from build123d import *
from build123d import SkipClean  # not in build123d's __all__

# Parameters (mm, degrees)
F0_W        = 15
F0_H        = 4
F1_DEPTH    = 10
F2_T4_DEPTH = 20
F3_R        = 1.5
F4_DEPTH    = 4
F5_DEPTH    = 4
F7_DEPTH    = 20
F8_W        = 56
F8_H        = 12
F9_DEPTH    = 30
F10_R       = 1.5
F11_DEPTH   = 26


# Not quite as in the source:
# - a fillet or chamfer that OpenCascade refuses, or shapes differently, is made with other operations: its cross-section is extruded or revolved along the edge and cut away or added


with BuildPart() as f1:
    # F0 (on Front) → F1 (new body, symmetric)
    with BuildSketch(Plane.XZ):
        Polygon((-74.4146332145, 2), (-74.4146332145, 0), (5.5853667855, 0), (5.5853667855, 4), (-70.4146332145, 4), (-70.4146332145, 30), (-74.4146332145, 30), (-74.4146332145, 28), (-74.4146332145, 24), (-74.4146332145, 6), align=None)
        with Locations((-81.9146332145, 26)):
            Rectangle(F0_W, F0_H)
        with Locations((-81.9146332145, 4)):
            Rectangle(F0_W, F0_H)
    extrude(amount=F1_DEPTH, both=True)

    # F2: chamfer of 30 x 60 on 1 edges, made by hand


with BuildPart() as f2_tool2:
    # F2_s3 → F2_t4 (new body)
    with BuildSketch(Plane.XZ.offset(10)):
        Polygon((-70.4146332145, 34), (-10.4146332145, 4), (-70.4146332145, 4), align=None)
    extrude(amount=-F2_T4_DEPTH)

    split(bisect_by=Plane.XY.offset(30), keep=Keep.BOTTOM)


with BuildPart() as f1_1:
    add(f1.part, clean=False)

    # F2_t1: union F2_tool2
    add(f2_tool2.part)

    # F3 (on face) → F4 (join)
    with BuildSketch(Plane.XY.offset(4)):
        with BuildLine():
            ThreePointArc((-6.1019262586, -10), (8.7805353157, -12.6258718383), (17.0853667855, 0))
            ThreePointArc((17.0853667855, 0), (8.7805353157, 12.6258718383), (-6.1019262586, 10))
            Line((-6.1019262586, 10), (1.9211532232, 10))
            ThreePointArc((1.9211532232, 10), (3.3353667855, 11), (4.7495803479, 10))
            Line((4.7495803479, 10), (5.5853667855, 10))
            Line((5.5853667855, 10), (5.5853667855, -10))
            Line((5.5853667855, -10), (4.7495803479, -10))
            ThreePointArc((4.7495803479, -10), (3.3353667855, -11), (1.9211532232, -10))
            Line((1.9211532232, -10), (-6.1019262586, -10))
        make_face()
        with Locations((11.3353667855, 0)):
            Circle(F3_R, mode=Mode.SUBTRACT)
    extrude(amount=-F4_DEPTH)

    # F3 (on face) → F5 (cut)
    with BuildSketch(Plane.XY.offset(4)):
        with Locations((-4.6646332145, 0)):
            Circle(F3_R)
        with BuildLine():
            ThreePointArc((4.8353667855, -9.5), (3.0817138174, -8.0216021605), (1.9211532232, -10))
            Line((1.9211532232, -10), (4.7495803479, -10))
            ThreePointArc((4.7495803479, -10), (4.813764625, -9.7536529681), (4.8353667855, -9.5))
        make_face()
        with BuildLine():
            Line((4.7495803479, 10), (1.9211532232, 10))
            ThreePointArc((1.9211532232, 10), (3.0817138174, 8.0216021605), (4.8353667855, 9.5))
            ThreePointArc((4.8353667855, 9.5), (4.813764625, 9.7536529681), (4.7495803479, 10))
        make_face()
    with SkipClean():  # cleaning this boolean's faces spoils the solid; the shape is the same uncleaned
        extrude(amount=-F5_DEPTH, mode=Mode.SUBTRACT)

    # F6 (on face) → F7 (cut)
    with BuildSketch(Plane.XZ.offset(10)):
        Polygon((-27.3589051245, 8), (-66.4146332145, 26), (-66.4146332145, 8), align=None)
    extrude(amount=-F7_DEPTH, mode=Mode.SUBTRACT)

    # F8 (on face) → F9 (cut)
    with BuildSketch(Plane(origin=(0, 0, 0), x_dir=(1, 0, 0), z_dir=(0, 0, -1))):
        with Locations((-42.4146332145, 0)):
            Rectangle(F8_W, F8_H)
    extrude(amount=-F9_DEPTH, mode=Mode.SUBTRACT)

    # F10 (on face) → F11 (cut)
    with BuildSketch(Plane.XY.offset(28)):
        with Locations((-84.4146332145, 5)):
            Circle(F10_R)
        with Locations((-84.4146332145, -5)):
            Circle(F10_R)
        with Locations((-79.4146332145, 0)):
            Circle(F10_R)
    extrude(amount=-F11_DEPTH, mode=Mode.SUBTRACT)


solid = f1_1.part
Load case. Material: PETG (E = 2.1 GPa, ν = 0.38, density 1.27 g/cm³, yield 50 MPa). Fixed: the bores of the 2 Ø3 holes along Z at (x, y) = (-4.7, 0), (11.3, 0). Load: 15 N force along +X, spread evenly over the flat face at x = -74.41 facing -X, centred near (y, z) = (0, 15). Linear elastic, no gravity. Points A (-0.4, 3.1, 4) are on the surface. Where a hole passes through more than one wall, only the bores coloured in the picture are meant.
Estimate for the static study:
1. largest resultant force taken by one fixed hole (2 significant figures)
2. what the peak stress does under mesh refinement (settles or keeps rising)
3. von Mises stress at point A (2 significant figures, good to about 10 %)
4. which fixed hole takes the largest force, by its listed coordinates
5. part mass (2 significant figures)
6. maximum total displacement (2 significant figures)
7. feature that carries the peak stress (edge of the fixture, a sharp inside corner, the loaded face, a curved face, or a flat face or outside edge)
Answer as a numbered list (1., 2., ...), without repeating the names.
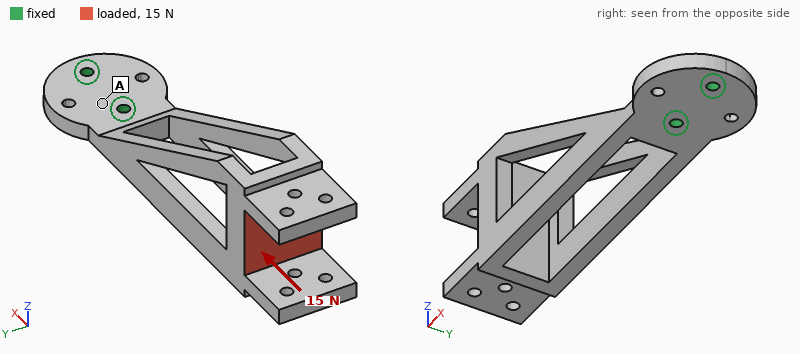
1. 12 N
2. keeps rising
3. 0.69 MPa
4. (-4.7, 0)
5. 17 g
6. 1.1 mm
7. edge of the fixture
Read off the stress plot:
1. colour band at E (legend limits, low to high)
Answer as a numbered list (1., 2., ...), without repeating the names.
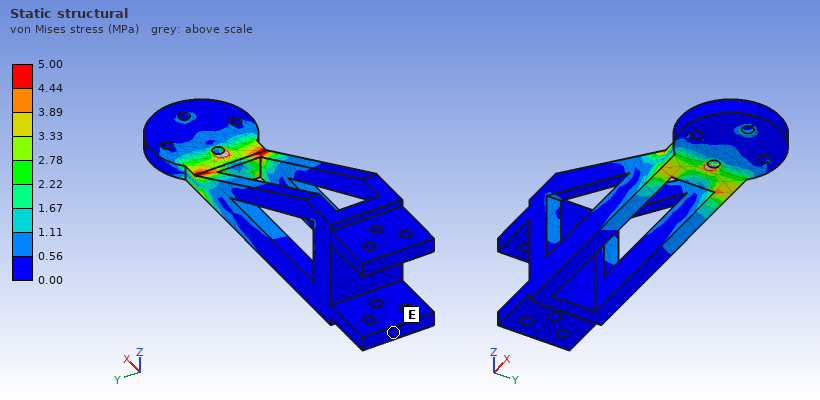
1. 0.00 to 0.56 MPa
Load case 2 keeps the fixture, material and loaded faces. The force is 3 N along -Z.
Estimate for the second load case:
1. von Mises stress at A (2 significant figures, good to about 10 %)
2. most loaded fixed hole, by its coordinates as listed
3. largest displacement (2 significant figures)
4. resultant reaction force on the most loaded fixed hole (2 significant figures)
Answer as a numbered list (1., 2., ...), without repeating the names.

1. 0.67 MPa
2. (-4.7, 0)
3. 1.1 mm
4. 8.3 N
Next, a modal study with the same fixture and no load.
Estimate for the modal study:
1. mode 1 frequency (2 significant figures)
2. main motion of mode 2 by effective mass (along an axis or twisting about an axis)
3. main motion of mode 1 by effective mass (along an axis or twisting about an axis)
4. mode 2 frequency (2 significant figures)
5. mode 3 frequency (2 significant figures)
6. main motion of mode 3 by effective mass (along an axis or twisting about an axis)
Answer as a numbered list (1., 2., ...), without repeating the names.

1. 95 Hz
2. along Y
3. along Z
4. 160 Hz
5. 360 Hz
6. twisting about X
